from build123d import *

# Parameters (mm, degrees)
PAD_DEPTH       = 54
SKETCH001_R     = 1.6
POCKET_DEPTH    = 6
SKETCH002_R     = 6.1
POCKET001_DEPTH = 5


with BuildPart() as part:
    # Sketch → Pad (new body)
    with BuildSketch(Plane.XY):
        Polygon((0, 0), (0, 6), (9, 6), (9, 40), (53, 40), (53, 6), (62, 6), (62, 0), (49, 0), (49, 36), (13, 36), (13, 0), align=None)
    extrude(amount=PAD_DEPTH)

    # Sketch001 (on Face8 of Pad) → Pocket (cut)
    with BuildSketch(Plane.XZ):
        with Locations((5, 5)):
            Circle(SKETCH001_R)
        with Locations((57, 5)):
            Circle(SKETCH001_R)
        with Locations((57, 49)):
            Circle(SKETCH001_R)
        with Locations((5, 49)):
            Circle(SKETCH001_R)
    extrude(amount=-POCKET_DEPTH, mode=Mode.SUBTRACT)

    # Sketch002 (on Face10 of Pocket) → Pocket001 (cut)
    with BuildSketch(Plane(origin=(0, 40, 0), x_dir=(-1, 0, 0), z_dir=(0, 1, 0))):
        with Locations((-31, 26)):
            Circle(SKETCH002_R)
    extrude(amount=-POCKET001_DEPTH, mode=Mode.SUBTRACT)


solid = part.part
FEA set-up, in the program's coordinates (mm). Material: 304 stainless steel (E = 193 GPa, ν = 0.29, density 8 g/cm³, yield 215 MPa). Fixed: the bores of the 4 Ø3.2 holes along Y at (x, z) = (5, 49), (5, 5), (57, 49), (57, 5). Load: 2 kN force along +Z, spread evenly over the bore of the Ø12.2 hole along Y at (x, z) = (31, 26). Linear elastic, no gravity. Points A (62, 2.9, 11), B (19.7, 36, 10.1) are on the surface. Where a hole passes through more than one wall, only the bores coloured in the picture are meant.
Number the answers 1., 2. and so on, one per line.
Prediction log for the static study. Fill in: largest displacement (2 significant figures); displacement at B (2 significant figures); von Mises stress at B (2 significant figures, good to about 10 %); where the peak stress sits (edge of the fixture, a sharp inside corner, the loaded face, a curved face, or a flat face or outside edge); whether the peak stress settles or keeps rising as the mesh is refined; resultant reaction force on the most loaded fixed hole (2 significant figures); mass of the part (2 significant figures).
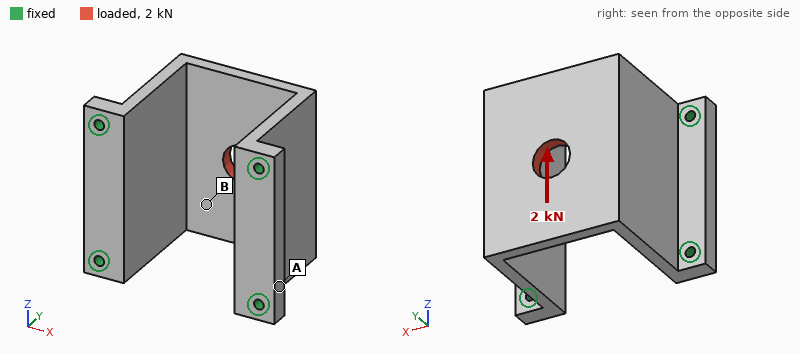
1. 8.7 µm
2. 7.4 µm
3. 9.5 MPa
4. edge of the fixture
5. keeps rising
6. 940 N
7. 240 g
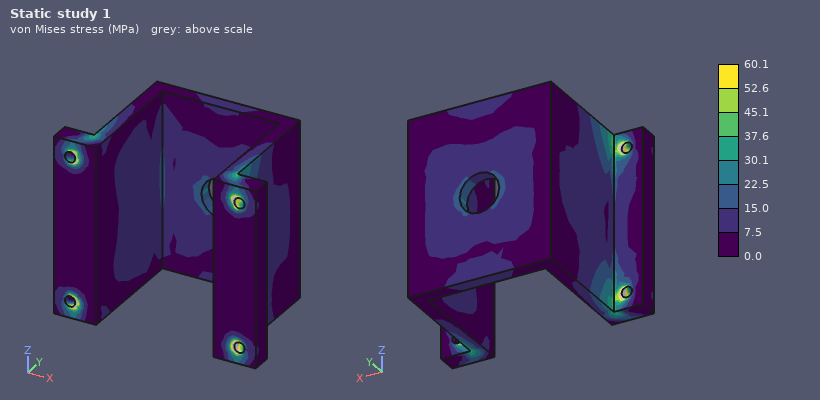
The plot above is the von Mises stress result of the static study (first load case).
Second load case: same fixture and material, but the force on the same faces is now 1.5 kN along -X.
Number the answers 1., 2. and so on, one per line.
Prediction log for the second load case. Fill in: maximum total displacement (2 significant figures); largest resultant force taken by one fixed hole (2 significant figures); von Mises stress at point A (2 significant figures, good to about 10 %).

1. 75 µm
2. 540 N
3. 44 MPa
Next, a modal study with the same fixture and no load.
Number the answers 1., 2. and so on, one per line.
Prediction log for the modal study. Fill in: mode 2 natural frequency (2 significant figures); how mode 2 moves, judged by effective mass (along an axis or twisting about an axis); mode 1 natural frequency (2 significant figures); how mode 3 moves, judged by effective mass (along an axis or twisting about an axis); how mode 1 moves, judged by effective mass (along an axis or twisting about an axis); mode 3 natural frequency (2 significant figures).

1. 6700 Hz
2. twisting about Y
3. 2200 Hz
4. along Z
5. along X
6. 7600 Hz
